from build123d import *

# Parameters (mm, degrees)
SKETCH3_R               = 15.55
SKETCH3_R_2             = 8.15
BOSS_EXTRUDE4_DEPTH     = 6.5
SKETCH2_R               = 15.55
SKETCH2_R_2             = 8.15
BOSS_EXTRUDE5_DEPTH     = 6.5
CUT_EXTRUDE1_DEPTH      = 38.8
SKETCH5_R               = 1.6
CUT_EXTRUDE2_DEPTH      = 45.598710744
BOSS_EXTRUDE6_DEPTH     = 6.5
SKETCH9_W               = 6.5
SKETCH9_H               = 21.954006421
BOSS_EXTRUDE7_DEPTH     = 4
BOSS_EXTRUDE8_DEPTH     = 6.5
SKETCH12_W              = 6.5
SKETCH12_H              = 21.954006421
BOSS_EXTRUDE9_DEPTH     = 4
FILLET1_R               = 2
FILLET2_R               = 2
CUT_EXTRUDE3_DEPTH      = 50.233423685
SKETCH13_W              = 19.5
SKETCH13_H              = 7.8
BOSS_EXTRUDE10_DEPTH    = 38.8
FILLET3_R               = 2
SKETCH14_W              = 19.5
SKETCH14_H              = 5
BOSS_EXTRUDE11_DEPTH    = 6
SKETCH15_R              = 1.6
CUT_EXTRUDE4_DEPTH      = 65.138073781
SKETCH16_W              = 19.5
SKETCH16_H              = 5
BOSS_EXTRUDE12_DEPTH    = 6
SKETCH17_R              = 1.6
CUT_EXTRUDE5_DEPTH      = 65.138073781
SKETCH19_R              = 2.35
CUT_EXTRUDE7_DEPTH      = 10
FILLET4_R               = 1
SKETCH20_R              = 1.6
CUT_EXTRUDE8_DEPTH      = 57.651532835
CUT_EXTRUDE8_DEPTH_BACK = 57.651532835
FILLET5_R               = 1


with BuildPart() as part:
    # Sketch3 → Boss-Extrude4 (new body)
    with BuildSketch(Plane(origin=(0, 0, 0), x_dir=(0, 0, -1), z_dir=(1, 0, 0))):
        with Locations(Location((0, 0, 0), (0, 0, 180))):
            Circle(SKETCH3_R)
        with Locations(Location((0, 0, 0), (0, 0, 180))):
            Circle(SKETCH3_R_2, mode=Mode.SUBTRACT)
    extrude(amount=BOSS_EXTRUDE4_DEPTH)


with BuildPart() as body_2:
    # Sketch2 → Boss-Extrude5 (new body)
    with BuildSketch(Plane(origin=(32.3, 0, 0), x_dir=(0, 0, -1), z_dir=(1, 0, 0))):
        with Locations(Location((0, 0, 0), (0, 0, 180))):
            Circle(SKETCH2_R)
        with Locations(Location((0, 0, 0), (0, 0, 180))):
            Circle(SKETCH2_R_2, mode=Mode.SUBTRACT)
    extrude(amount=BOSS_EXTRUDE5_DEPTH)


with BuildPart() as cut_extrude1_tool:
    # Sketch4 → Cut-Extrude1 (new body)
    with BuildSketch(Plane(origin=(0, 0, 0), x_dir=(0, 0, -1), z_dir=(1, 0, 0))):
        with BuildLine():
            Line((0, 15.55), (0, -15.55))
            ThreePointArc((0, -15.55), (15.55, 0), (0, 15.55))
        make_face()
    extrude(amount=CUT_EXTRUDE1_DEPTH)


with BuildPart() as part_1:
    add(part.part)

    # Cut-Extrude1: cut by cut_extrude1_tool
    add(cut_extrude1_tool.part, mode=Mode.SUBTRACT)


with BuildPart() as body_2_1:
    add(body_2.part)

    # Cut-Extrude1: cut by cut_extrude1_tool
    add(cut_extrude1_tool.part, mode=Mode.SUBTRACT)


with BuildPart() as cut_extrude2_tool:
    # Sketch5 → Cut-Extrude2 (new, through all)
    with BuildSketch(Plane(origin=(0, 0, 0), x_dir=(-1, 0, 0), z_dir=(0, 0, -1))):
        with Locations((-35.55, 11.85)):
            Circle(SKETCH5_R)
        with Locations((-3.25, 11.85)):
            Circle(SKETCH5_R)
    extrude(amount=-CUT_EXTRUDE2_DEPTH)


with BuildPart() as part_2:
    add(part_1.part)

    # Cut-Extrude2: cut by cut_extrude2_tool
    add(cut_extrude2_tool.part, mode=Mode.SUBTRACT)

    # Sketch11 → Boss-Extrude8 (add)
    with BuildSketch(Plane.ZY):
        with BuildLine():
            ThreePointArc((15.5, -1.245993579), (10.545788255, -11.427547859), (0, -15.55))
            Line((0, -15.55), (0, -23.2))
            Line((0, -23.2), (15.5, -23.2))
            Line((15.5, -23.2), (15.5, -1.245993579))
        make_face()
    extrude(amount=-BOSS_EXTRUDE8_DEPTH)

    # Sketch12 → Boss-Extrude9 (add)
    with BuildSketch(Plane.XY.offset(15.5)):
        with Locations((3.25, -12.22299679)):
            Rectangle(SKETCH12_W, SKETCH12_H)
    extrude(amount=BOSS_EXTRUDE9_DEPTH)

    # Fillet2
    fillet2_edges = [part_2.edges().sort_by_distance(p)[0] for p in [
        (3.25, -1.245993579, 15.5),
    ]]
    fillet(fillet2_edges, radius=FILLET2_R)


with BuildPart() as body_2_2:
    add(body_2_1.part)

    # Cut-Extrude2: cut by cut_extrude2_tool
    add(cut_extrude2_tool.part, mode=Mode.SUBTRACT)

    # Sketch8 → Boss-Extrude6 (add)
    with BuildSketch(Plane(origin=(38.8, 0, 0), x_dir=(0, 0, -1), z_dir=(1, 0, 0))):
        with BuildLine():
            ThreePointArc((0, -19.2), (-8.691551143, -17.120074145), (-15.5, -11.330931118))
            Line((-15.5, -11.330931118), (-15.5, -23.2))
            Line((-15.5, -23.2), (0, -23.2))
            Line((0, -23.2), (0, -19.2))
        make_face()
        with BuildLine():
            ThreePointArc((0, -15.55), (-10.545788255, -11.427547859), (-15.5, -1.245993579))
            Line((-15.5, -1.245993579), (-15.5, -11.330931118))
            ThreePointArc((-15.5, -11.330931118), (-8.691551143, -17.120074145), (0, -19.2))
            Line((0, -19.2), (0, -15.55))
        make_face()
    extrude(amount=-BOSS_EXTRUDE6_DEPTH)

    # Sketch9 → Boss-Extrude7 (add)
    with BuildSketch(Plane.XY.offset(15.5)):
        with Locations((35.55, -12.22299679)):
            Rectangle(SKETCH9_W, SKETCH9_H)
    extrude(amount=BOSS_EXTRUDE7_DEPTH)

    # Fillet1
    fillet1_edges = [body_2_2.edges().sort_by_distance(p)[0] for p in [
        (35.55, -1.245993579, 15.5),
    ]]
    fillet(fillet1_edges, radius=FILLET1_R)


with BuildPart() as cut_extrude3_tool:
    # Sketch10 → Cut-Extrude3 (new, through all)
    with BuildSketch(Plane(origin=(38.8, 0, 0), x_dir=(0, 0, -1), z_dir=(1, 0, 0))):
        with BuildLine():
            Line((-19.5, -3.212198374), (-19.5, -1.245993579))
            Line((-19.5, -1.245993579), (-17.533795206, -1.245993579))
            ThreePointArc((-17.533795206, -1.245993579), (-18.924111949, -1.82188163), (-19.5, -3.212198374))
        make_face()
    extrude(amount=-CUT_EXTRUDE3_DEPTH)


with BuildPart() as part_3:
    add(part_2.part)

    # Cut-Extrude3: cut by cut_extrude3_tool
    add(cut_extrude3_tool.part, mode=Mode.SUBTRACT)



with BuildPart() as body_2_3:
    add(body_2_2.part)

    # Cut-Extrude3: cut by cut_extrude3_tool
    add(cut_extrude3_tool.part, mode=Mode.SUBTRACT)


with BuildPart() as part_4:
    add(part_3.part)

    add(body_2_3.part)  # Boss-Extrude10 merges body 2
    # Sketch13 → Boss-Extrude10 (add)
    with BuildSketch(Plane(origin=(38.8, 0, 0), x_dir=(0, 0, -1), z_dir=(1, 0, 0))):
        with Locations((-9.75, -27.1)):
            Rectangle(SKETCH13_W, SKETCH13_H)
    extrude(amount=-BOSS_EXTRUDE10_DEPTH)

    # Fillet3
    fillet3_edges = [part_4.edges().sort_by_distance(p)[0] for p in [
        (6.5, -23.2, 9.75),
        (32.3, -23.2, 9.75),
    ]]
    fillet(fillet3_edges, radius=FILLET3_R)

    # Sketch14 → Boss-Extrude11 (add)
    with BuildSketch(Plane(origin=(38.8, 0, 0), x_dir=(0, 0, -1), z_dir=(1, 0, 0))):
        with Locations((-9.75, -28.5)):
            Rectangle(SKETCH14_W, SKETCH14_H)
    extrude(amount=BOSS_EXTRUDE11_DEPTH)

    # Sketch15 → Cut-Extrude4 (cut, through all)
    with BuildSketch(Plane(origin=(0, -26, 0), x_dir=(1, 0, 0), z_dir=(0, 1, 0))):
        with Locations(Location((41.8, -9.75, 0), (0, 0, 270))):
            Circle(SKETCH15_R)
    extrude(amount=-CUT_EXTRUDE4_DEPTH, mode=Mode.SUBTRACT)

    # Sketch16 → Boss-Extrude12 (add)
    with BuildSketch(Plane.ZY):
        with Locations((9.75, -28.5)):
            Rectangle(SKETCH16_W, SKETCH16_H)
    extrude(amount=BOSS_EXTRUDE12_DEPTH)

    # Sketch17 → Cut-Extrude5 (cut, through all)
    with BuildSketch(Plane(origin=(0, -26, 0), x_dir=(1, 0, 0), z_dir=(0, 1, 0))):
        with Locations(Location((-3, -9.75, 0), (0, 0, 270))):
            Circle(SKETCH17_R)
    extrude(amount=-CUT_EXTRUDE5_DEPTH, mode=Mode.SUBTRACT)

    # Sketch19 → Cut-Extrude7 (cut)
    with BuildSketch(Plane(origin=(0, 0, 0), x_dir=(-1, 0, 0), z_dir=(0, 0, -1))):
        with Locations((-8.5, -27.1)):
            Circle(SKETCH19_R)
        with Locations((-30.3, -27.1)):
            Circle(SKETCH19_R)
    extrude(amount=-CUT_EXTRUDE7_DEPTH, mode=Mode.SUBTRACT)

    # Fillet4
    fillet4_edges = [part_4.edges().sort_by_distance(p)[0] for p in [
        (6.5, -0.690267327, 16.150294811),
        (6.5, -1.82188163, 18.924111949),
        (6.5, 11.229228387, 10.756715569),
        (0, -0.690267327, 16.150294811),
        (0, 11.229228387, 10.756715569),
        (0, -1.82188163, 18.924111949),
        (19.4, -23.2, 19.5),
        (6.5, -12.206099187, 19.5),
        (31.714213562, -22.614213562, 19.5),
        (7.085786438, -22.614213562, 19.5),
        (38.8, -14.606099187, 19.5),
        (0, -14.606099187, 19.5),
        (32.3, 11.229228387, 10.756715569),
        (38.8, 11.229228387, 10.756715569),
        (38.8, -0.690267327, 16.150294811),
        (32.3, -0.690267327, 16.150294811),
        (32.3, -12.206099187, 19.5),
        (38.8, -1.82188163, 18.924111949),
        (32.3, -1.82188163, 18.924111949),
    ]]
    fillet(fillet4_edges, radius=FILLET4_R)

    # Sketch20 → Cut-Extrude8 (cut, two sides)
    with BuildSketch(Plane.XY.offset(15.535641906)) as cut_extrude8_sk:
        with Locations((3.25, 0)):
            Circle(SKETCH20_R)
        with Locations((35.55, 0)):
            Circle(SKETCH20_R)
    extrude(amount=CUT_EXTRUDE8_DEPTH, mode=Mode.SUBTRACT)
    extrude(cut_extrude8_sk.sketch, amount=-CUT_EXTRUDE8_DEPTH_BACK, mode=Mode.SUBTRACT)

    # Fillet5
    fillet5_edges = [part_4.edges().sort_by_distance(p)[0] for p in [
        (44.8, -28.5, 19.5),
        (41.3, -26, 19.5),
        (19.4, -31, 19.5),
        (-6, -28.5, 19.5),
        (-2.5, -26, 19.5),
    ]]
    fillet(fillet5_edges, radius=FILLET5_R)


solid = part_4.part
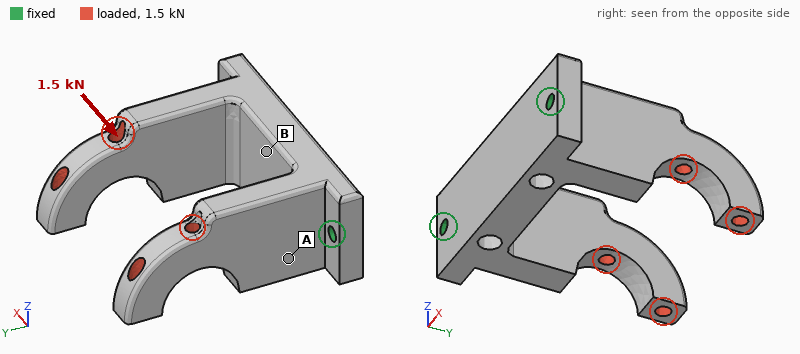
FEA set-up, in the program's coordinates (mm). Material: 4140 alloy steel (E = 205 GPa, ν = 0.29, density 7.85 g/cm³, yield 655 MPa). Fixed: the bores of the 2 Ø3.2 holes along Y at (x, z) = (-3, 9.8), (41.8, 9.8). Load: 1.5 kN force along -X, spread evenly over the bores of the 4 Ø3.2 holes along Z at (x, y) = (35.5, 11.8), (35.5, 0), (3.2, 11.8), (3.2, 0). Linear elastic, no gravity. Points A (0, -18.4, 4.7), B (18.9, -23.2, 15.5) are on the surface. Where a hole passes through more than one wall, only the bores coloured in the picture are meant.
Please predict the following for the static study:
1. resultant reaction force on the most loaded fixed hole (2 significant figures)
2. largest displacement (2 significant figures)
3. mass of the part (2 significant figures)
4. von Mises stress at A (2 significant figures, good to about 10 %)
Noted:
1.4 kN
0.20 mm
100 g
120 MPa
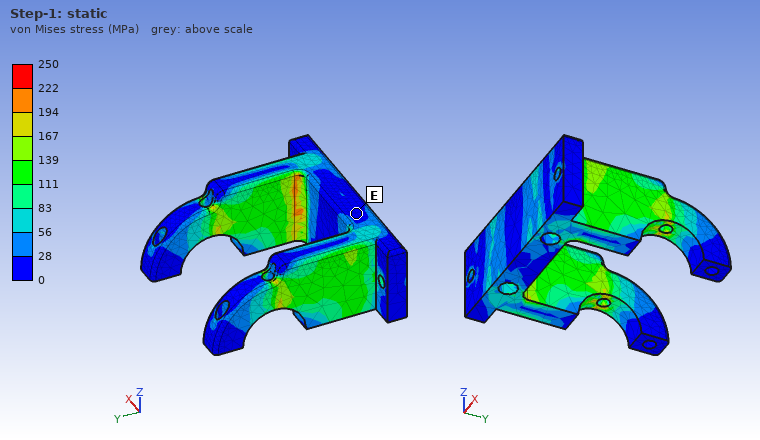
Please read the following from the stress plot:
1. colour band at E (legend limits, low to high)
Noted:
0 to 28 MPa
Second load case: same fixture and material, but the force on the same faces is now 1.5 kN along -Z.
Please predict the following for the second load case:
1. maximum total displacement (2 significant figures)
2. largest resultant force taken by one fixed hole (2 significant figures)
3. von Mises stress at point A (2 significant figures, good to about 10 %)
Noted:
0.18 mm
760 N
38 MPa
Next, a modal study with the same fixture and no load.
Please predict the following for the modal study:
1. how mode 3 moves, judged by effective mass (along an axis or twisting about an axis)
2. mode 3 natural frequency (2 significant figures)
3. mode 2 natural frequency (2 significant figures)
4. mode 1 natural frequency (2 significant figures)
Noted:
along X
4200 Hz
3700 Hz
3600 Hz
